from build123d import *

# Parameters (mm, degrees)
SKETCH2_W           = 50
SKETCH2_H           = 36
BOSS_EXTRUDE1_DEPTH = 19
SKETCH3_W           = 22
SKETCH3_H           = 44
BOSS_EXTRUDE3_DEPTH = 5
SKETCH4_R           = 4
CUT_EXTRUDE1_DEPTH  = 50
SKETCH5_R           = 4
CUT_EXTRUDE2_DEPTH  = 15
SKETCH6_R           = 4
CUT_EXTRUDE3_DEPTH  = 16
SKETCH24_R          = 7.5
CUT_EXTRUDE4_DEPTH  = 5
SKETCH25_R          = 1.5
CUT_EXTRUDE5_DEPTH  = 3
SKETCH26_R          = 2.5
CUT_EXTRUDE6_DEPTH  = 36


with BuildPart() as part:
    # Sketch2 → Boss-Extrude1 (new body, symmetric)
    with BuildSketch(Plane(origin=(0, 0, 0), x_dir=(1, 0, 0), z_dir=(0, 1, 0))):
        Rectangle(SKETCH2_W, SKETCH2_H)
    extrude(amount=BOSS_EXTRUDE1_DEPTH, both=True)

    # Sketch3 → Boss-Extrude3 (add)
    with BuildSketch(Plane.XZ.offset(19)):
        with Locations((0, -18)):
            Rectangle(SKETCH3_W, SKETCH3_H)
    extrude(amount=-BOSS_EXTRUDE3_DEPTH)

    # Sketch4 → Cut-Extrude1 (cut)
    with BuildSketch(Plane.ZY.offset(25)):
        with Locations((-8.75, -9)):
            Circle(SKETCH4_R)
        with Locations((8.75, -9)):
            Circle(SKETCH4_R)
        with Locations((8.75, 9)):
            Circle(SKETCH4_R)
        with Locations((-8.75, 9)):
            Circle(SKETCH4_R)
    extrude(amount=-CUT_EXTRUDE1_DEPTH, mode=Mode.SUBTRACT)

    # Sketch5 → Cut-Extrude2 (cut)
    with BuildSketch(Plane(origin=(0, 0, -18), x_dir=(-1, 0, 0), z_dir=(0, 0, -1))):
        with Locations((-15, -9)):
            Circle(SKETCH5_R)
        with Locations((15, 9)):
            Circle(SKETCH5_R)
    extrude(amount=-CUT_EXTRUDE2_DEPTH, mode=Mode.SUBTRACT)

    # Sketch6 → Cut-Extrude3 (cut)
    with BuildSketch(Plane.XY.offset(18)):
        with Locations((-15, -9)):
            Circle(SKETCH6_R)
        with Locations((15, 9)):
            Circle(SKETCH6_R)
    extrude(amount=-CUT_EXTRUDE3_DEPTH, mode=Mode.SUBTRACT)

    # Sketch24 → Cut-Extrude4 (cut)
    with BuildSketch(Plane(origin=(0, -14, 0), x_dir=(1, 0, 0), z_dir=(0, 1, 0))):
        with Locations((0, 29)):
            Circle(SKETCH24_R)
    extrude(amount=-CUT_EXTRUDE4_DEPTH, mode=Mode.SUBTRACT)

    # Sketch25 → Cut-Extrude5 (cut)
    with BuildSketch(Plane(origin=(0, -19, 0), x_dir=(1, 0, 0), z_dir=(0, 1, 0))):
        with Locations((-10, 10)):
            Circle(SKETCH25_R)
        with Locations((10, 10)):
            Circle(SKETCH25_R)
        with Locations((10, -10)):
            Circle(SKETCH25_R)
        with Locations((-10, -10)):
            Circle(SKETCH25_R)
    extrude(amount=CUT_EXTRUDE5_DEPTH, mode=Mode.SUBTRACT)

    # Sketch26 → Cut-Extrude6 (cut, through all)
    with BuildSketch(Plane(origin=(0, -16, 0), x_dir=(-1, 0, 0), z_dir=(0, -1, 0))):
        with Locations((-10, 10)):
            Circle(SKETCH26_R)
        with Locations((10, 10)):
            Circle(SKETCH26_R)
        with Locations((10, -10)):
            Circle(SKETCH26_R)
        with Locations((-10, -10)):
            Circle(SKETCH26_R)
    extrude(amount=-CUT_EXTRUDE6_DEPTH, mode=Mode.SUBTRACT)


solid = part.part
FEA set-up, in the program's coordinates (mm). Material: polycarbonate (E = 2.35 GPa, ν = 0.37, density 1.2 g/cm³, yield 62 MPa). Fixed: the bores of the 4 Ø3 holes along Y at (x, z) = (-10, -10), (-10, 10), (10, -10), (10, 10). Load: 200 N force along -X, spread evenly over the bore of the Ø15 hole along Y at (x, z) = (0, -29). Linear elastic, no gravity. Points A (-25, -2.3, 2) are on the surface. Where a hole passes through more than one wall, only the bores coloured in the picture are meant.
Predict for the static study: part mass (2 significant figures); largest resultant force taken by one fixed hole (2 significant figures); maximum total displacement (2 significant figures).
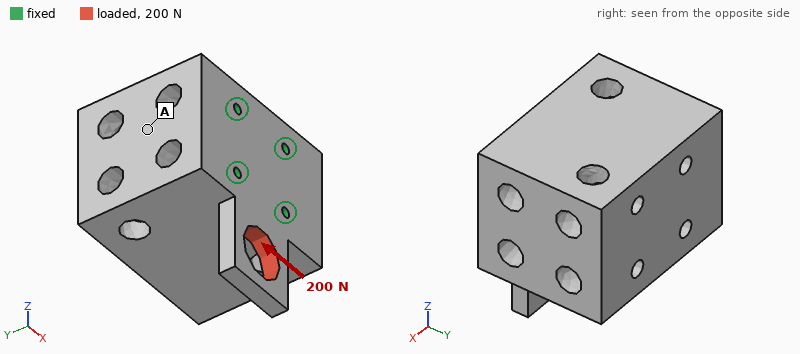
68 g
160 N
0.28 mm
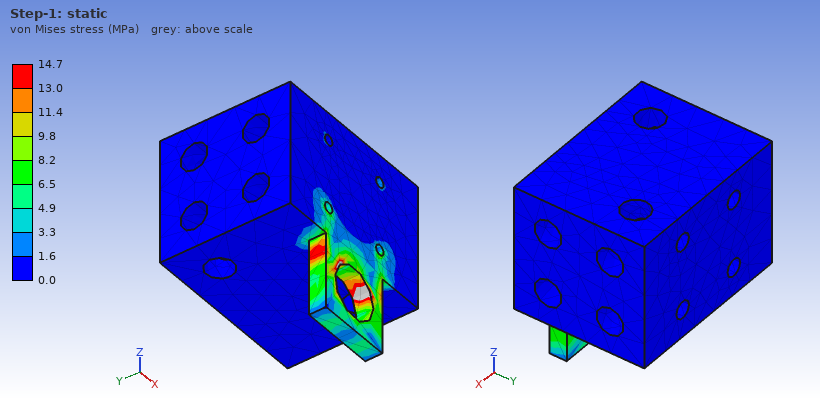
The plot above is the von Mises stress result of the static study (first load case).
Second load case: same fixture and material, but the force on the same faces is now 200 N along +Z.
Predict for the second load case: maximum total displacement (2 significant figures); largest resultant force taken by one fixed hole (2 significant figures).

61 µm
78 N
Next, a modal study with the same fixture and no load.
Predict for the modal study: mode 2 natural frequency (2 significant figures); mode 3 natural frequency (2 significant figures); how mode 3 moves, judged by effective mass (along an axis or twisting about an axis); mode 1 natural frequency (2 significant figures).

1400 Hz
1700 Hz
along Z
1400 Hz
